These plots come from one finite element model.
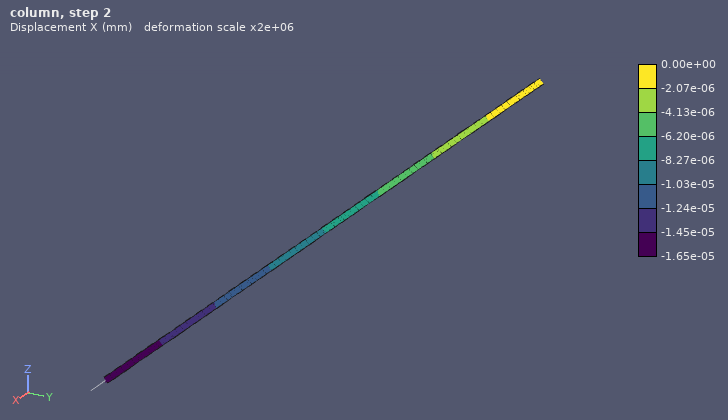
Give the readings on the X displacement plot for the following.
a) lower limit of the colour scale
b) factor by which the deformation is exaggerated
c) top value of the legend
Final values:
-1.65e-05 mm
2e+06
0.00e+00 mm
